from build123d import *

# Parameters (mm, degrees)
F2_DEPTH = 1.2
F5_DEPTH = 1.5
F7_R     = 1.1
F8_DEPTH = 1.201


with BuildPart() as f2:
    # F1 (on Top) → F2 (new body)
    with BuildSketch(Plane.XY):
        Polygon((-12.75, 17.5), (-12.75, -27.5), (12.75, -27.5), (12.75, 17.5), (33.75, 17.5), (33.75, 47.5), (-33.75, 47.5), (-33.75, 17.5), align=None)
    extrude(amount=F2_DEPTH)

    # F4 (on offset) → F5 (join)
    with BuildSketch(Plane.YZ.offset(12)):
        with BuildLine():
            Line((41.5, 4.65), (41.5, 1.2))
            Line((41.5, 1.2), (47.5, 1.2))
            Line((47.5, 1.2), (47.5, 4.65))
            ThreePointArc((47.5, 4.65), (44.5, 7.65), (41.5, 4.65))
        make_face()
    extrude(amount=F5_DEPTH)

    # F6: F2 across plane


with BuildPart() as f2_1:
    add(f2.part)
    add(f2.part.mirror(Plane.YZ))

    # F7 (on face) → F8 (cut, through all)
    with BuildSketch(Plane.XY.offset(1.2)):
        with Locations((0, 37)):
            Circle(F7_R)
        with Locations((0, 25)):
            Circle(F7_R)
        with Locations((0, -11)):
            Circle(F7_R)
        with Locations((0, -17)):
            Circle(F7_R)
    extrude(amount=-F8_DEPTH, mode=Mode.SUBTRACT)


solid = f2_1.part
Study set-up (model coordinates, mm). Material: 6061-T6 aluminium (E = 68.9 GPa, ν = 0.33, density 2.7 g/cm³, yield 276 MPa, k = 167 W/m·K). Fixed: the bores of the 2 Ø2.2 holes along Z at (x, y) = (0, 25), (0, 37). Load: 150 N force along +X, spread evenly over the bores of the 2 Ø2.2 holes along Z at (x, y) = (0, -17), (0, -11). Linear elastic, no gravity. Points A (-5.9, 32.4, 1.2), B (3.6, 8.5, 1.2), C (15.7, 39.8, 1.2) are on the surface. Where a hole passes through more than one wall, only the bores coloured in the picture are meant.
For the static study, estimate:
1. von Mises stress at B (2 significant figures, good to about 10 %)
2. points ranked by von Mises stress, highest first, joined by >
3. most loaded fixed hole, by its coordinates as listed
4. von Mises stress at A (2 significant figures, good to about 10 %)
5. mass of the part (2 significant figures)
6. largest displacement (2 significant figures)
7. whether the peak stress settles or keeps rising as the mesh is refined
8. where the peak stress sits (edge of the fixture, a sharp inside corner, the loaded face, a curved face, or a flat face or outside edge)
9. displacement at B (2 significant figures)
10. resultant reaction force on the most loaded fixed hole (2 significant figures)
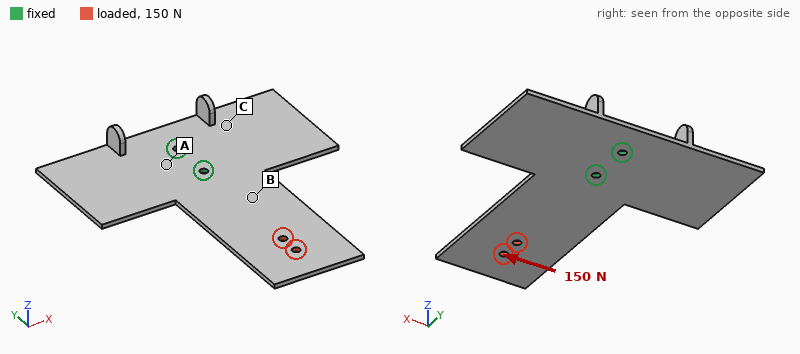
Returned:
13 MPa
A > B > C
(0, 25)
26 MPa
11 g
96 µm
keeps rising
edge of the fixture
25 µm
580 N
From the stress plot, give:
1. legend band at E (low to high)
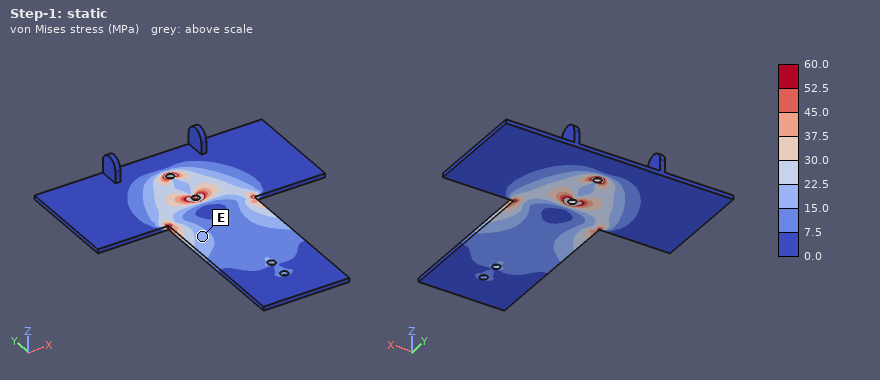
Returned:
15.0 to 22.5 MPa
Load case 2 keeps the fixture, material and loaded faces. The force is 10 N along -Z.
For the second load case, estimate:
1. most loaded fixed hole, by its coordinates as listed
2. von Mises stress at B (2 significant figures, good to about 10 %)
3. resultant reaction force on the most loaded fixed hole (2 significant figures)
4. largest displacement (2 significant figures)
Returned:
(0, 25)
34 MPa
25 N
1.1 mm
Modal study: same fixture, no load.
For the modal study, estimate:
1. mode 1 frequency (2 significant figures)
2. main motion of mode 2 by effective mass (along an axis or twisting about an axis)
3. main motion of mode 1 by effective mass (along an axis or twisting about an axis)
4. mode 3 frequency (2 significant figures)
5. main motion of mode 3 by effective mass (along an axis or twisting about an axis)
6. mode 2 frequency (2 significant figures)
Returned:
370 Hz
twisting about Y
along Z
970 Hz
along Z
840 Hz
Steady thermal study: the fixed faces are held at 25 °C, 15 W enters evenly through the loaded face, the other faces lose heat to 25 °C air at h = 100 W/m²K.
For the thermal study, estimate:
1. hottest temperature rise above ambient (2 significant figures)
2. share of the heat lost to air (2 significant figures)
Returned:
67 K
70 %
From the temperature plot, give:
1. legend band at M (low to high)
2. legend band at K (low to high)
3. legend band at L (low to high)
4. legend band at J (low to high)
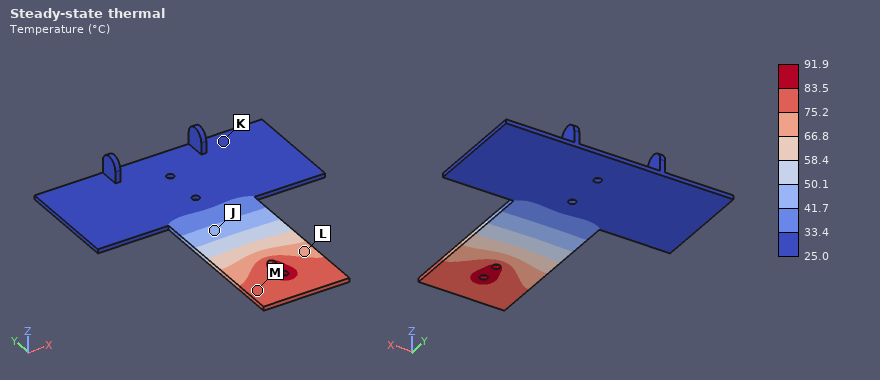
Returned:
75.2 to 83.5 °C
25.0 to 33.4 °C
66.8 to 75.2 °C
41.7 to 50.1 °C
